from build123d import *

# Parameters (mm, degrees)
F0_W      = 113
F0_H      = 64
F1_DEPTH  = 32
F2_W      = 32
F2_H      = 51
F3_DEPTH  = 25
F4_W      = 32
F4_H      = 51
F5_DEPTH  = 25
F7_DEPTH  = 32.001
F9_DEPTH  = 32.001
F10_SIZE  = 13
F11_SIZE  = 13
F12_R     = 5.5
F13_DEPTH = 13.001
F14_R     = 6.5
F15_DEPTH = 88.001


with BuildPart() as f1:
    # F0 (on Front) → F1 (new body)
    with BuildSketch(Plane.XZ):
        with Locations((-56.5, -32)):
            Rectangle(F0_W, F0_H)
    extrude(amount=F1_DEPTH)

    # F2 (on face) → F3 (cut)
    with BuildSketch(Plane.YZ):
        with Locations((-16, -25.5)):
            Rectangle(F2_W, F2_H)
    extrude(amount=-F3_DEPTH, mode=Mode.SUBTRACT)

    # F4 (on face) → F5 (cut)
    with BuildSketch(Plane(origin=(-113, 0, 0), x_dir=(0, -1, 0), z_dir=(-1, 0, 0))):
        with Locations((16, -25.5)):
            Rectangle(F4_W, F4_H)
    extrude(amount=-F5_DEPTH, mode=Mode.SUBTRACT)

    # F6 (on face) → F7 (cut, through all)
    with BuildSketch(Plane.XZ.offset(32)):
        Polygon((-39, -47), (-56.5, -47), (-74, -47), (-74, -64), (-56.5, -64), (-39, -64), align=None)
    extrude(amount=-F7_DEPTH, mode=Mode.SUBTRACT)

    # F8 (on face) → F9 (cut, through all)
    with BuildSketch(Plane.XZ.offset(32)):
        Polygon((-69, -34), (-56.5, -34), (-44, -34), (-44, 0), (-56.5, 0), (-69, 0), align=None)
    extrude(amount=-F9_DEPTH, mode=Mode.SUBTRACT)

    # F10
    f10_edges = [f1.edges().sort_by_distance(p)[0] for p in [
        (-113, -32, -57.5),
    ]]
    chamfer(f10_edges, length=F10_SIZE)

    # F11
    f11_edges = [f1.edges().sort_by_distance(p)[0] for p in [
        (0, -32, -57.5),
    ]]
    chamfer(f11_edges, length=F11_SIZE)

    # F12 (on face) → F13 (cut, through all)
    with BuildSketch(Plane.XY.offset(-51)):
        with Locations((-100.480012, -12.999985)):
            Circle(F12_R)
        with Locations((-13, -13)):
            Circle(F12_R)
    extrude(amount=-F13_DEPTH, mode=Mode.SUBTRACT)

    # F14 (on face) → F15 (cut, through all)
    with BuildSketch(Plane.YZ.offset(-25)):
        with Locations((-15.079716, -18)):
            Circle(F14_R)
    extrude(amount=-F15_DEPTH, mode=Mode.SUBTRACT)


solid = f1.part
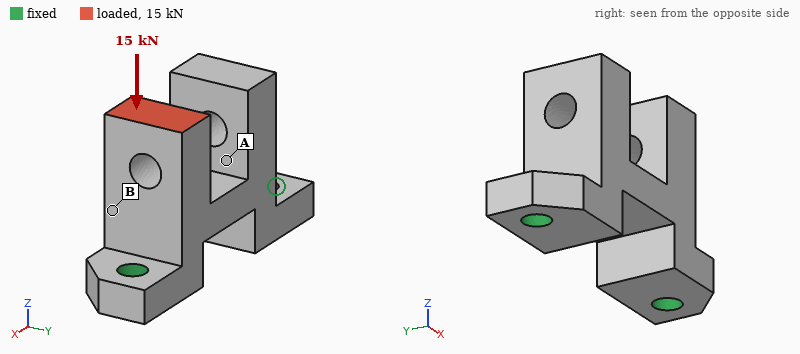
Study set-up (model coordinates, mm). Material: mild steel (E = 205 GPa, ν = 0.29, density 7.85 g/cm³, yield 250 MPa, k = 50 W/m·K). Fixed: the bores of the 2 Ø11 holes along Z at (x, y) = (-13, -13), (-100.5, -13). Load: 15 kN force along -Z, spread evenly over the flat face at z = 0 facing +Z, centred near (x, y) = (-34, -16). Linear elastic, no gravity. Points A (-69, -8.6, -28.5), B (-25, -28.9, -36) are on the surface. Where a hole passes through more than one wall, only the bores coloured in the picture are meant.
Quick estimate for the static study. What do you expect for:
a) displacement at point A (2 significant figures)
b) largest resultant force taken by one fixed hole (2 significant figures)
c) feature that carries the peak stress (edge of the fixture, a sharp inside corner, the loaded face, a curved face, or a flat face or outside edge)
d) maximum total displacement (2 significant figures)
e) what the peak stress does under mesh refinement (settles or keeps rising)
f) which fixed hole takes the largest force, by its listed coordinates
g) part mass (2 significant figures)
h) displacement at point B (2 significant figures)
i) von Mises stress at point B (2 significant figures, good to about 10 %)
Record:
5.2 µm
13 kN
edge of the fixture
25 µm
keeps rising
(-13, -13)
740 g
18 µm
38 MPa
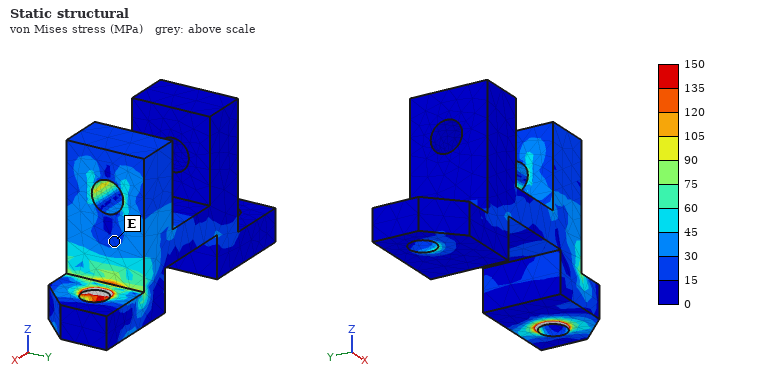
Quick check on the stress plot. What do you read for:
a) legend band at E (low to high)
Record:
15 to 30 MPa
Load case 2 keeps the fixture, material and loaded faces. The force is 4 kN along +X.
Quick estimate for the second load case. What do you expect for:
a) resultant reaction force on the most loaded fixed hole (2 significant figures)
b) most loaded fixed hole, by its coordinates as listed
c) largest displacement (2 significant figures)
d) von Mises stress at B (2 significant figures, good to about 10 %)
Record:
6.1 kN
(-100.5, -13)
59 µm
66 MPa
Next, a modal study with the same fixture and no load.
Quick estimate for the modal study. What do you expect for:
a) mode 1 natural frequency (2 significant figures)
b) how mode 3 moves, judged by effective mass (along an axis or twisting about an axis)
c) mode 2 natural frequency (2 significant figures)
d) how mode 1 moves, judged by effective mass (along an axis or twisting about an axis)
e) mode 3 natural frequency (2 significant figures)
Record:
2700 Hz
along X
4500 Hz
along Y
5500 Hz
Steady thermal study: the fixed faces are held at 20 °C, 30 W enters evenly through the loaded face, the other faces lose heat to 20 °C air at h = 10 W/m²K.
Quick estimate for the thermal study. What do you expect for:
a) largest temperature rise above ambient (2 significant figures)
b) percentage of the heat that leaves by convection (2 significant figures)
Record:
71 K
12 %
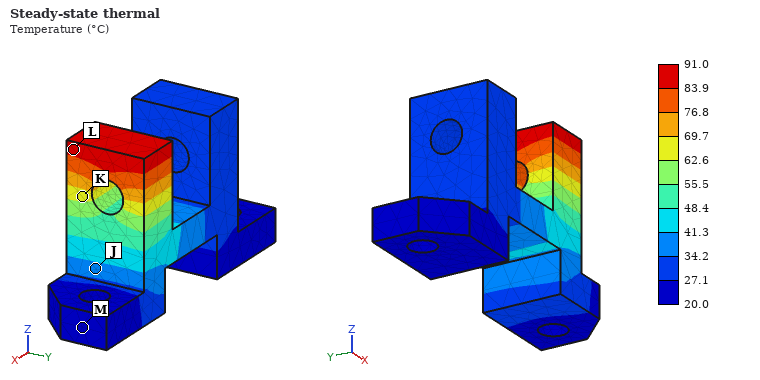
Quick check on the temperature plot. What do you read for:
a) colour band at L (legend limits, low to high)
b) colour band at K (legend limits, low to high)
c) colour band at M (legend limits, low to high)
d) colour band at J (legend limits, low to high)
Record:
83.9 to 91.0 °C
62.6 to 69.7 °C
20.0 to 27.1 °C
34.2 to 41.3 °C
